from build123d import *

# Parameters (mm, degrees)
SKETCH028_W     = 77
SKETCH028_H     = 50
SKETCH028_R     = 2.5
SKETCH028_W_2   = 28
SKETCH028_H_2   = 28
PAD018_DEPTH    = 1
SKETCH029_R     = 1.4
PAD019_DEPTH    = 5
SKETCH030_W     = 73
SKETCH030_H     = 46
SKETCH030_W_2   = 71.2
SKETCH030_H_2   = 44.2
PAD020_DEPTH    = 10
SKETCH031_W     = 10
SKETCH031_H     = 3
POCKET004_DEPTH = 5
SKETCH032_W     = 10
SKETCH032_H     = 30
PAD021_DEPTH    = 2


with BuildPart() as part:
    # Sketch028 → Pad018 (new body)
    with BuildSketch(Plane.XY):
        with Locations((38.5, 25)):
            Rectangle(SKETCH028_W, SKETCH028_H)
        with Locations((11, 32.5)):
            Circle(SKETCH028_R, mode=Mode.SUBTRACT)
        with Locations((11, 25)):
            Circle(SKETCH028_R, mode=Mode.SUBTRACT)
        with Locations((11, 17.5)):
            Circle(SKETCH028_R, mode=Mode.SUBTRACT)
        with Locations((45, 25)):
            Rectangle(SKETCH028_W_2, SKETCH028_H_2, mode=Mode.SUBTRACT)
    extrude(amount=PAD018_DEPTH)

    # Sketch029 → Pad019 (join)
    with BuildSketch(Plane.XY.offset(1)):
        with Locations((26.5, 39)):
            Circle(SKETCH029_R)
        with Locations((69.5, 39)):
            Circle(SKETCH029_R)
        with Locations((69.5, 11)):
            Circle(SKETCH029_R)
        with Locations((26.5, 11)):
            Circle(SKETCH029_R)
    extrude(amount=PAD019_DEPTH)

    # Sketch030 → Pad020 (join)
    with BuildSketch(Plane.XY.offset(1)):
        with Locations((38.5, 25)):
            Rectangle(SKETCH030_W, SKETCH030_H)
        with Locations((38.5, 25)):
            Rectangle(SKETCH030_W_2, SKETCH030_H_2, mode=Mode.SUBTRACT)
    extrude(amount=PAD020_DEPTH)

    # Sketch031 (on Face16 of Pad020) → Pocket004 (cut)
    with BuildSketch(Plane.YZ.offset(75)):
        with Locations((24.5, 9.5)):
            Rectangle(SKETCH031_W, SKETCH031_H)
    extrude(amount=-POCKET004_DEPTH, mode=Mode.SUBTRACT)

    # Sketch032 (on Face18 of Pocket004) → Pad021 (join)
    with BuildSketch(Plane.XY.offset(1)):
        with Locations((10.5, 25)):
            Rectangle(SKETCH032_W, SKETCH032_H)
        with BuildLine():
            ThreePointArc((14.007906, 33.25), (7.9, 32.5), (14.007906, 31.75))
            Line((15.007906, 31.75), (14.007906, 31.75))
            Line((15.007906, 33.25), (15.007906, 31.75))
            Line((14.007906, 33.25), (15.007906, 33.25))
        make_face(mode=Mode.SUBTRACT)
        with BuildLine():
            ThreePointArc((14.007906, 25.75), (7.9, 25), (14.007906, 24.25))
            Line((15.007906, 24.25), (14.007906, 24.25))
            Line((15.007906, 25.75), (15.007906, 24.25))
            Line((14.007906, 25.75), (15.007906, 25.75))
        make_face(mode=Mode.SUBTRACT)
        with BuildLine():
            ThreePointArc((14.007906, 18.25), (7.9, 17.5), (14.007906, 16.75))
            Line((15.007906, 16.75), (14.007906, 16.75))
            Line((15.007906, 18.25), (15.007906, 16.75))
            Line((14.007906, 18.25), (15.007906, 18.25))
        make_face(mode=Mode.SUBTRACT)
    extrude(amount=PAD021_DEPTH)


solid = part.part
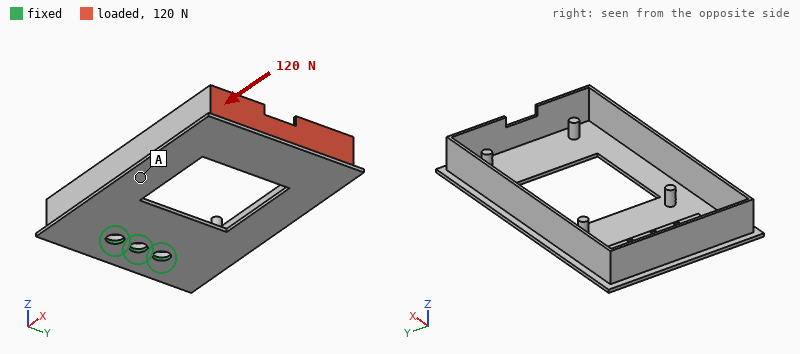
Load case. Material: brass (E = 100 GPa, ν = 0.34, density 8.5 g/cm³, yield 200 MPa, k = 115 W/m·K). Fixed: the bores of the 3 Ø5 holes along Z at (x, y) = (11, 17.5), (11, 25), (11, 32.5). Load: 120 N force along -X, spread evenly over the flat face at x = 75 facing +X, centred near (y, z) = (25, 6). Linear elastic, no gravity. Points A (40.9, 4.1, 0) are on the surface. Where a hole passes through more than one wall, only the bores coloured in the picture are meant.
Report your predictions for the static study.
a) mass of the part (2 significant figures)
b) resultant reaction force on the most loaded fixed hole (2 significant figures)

48 g
62 N
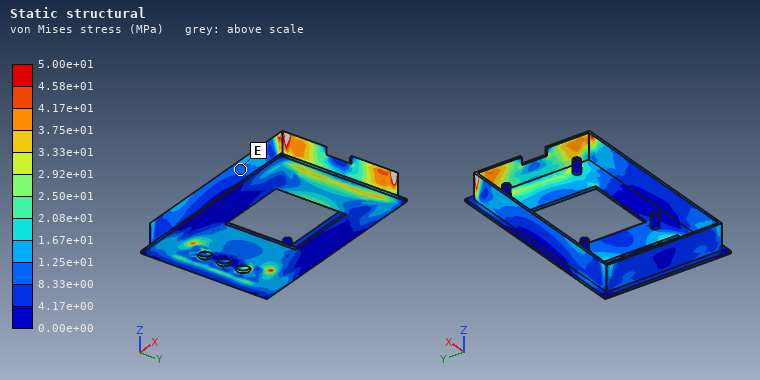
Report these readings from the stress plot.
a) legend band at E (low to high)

8.33e+00 to 1.25e+01 MPa
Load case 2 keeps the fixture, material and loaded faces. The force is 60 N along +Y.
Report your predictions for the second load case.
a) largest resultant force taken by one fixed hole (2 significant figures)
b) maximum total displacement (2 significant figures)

200 N
0.33 mm
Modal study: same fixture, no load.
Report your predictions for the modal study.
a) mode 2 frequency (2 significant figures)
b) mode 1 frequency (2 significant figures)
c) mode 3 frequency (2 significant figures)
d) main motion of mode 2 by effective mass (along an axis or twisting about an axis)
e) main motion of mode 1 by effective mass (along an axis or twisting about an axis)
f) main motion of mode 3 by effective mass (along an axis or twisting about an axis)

380 Hz
280 Hz
1700 Hz
twisting about X
along Z
along Y
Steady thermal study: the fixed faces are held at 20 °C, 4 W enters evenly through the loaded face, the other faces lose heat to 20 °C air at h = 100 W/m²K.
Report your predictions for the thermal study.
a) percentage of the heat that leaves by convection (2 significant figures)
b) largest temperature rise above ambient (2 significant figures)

94 %
14 K
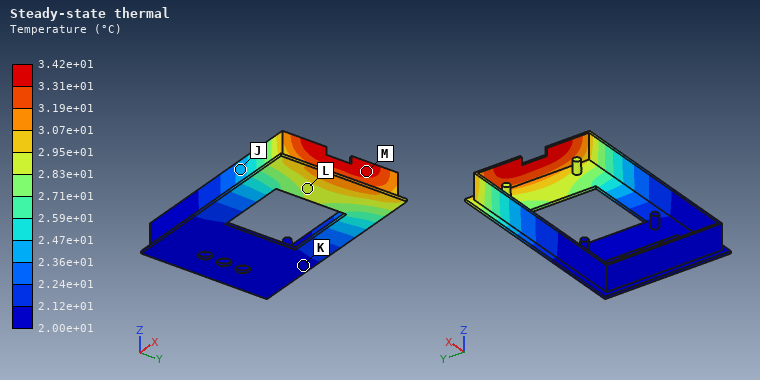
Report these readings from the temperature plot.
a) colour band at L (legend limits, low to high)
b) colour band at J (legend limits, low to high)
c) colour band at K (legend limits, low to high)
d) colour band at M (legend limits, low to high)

2.83e+01 to 2.95e+01 °C
2.36e+01 to 2.47e+01 °C
2.00e+01 to 2.12e+01 °C
3.31e+01 to 3.42e+01 °C
